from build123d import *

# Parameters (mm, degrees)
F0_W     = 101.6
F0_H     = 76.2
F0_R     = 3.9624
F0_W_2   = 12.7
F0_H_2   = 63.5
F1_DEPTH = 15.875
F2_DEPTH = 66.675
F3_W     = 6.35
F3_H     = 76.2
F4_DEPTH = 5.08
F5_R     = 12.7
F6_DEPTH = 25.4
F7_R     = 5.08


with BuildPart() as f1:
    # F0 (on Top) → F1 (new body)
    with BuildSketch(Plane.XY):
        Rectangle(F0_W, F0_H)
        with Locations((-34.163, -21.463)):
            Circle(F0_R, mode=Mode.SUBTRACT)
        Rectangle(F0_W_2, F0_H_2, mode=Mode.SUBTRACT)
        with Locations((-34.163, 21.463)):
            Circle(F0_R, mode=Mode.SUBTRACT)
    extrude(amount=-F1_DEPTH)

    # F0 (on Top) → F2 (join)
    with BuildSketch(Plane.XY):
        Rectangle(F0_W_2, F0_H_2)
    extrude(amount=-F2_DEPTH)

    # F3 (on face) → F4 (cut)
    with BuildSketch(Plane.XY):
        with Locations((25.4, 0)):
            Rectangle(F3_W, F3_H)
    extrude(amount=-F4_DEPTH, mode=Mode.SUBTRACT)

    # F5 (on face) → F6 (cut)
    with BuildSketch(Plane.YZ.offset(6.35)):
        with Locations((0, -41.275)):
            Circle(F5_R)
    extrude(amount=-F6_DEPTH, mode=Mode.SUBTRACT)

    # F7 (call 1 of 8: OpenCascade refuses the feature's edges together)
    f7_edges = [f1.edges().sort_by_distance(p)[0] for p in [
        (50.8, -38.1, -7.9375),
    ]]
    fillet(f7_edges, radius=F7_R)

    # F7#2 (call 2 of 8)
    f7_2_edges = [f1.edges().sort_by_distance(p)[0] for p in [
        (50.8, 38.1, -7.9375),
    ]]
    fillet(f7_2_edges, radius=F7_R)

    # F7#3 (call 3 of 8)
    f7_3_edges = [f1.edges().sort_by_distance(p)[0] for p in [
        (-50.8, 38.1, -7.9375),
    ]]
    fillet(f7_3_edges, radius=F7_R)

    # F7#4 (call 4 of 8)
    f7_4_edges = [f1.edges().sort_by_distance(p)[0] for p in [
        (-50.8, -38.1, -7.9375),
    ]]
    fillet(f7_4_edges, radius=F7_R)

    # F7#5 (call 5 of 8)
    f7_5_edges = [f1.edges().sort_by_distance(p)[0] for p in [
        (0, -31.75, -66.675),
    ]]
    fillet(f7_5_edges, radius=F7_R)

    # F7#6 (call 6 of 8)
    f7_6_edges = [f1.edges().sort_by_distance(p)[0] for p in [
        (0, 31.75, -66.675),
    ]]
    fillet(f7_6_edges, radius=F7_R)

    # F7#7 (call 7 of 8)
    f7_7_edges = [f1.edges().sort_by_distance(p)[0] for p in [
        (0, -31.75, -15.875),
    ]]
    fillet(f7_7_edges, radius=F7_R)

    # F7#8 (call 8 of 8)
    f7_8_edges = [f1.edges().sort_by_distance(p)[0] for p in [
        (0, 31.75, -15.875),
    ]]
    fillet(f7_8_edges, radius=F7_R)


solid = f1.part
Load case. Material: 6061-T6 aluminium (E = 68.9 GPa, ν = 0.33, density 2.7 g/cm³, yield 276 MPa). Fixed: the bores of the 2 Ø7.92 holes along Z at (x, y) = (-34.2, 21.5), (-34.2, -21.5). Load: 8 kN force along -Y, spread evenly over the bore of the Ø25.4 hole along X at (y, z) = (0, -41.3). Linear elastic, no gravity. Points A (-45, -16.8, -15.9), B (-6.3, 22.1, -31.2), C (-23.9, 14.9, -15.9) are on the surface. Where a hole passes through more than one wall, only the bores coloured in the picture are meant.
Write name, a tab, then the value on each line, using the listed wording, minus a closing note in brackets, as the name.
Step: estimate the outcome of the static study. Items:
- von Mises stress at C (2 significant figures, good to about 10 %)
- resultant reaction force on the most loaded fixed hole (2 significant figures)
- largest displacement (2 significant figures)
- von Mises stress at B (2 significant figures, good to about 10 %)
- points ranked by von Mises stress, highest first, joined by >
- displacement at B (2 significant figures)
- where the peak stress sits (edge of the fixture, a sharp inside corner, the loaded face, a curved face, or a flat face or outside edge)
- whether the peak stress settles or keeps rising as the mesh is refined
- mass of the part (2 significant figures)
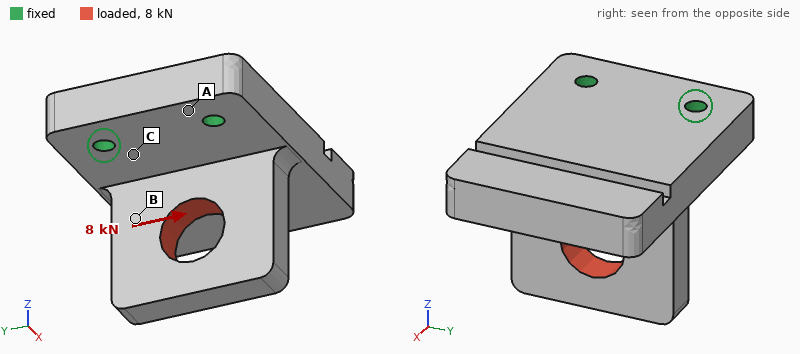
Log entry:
von Mises stress at C	47 MPa
resultant reaction force on the most loaded fixed hole	8.4 kN
largest displacement	0.16 mm
von Mises stress at B	29 MPa
points ranked by von Mises stress, highest first, joined by >	C > B > A
displacement at B	0.072 mm
where the peak stress sits	edge of the fixture
whether the peak stress settles or keeps rising as the mesh is refined	keeps rising
mass of the part	410 g
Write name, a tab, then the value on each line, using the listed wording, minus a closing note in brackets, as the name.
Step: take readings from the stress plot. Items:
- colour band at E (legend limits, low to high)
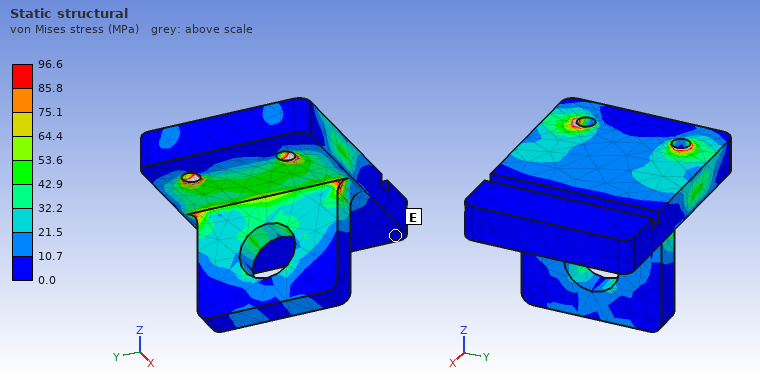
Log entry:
colour band at E	0.0 to 10.7 MPa
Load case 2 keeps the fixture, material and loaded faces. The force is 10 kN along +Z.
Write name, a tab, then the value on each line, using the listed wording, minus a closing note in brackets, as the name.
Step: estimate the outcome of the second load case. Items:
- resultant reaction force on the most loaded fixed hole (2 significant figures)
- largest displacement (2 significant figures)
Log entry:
resultant reaction force on the most loaded fixed hole	5.0 kN
largest displacement	0.29 mm
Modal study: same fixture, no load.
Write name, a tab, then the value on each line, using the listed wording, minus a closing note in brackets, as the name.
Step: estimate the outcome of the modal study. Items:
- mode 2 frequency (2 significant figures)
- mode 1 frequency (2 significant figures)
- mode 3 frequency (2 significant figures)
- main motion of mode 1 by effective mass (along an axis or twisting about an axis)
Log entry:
mode 2 frequency	3300 Hz
mode 1 frequency	1500 Hz
mode 3 frequency	3500 Hz
main motion of mode 1 by effective mass	along Z
